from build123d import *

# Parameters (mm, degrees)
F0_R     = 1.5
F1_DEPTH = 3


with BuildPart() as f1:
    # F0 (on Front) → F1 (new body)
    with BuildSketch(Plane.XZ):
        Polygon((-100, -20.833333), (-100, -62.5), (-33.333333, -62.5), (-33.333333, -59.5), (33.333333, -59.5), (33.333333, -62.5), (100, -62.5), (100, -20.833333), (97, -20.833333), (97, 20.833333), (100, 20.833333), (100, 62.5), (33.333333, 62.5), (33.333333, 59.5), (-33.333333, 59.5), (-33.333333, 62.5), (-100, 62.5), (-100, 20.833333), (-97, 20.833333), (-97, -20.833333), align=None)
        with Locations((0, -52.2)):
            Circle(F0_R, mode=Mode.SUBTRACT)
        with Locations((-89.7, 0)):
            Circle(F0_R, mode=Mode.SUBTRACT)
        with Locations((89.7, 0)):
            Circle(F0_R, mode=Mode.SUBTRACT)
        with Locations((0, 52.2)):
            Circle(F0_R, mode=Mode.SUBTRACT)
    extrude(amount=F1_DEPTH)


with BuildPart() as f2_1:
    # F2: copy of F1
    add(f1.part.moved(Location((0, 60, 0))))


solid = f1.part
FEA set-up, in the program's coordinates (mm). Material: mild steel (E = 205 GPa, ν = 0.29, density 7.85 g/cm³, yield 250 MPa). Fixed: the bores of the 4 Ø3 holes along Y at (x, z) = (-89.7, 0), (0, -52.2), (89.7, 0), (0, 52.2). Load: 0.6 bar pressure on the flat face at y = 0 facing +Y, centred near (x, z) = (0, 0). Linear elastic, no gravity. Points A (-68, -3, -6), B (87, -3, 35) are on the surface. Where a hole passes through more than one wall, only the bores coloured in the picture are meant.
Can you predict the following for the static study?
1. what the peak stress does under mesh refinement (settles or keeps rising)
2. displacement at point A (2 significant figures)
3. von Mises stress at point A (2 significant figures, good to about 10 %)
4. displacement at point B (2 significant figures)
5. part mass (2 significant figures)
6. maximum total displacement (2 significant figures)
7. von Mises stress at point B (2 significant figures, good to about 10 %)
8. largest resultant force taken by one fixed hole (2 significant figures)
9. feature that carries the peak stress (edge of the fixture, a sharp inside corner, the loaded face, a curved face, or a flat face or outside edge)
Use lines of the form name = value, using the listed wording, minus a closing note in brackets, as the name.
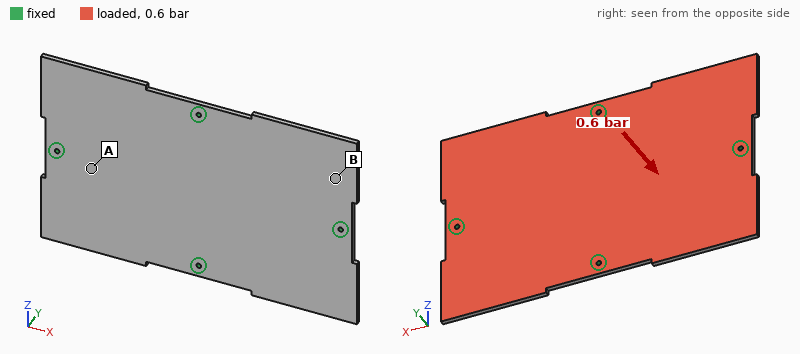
what the peak stress does under mesh refinement = keeps rising
displacement at point A = 0.034 mm
von Mises stress at point A = 32 MPa
displacement at point B = 0.072 mm
part mass = 570 g
maximum total displacement = 0.15 mm
von Mises stress at point B = 14 MPa
largest resultant force taken by one fixed hole = 370 N
feature that carries the peak stress = edge of the fixture
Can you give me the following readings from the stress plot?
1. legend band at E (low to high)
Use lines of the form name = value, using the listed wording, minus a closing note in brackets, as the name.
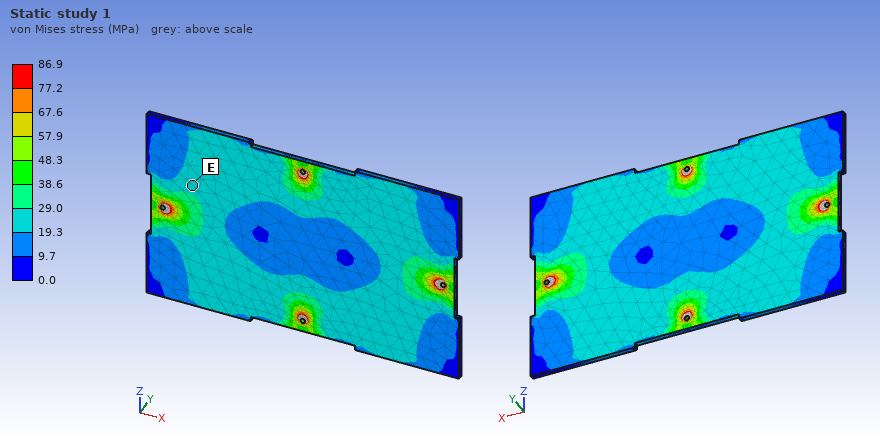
legend band at E = 19.3 to 29.0 MPa
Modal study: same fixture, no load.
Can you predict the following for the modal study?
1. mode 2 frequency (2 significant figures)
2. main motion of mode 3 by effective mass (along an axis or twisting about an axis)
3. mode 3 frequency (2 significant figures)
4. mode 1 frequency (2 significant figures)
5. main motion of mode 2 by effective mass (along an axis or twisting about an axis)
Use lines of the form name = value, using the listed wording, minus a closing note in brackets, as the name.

mode 2 frequency = 730 Hz
main motion of mode 3 by effective mass = twisting about Z
mode 3 frequency = 810 Hz
mode 1 frequency = 700 Hz
main motion of mode 2 by effective mass = twisting about X
